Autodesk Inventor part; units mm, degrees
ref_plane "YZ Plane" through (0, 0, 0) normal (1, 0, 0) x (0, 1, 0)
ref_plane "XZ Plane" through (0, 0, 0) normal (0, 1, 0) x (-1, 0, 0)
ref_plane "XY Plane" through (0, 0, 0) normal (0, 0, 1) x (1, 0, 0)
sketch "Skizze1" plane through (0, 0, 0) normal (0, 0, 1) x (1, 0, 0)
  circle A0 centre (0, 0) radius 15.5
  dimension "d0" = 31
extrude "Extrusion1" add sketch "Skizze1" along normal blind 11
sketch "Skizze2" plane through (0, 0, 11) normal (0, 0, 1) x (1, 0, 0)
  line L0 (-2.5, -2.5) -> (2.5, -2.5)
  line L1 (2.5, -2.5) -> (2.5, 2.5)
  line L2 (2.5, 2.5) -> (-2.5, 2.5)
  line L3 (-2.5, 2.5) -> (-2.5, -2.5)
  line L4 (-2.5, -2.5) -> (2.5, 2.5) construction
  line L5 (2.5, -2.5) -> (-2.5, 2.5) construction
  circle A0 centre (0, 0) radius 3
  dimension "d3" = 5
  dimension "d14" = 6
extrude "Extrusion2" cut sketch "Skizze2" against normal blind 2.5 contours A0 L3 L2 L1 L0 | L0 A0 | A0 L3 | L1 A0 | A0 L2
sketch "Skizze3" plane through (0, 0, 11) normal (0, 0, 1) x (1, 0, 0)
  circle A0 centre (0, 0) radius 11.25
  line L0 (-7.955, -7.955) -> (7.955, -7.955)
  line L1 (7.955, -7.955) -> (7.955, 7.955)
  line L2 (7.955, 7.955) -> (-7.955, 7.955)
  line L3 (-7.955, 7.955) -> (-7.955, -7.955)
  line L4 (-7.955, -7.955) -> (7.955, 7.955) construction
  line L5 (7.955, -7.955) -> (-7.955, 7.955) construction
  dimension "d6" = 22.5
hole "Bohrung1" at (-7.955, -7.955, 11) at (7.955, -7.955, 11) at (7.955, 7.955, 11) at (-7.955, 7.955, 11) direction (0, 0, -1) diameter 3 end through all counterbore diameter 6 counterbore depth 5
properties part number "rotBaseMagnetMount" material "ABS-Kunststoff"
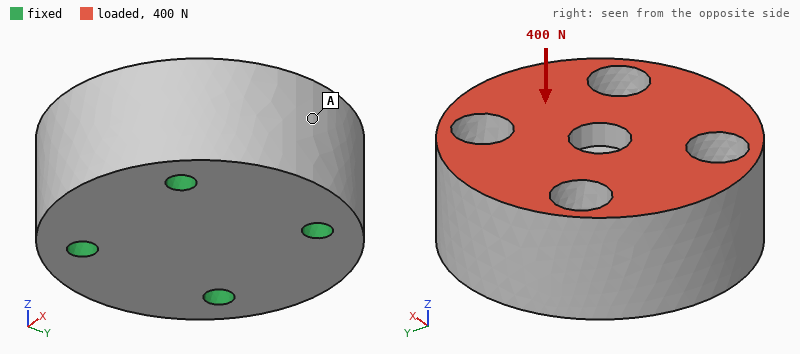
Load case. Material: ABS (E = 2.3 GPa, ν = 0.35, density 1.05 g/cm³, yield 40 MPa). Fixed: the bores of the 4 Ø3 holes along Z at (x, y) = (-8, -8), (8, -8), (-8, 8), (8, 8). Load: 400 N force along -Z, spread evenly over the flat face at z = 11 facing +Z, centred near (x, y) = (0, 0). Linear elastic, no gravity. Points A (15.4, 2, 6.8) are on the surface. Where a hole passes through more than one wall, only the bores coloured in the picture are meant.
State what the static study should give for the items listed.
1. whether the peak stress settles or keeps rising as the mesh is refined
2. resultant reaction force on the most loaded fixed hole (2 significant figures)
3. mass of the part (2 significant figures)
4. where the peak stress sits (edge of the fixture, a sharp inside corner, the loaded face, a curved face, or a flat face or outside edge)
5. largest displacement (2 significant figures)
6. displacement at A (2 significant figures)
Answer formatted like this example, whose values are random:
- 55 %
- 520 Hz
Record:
- keeps rising
- 100 N
- 7.9 g
- edge of the fixture
- 8.8 µm
- 7.5 µm
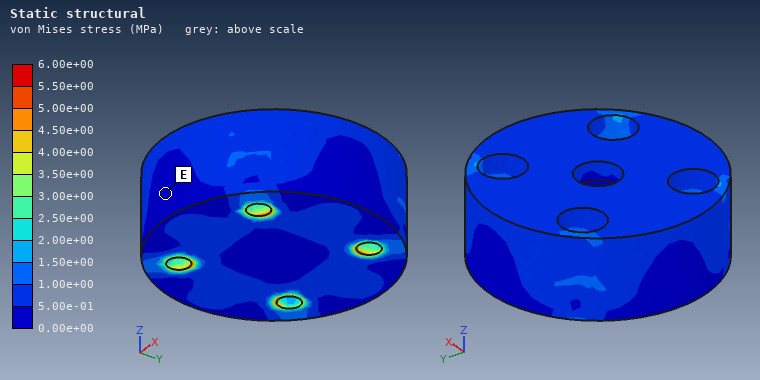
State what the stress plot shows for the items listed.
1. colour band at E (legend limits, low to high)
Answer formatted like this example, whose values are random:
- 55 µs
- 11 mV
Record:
- 0.00e+00 to 5.00e-01 MPa
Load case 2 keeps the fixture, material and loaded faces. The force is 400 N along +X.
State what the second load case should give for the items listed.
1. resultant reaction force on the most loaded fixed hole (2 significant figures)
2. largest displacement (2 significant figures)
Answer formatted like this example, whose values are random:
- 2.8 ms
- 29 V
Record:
- 130 N
- 25 µm
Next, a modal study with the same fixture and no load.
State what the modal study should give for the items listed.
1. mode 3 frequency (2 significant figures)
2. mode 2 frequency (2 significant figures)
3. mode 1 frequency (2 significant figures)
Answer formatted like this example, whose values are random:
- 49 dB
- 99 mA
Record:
- 15 kHz
- 14 kHz
- 14 kHz
